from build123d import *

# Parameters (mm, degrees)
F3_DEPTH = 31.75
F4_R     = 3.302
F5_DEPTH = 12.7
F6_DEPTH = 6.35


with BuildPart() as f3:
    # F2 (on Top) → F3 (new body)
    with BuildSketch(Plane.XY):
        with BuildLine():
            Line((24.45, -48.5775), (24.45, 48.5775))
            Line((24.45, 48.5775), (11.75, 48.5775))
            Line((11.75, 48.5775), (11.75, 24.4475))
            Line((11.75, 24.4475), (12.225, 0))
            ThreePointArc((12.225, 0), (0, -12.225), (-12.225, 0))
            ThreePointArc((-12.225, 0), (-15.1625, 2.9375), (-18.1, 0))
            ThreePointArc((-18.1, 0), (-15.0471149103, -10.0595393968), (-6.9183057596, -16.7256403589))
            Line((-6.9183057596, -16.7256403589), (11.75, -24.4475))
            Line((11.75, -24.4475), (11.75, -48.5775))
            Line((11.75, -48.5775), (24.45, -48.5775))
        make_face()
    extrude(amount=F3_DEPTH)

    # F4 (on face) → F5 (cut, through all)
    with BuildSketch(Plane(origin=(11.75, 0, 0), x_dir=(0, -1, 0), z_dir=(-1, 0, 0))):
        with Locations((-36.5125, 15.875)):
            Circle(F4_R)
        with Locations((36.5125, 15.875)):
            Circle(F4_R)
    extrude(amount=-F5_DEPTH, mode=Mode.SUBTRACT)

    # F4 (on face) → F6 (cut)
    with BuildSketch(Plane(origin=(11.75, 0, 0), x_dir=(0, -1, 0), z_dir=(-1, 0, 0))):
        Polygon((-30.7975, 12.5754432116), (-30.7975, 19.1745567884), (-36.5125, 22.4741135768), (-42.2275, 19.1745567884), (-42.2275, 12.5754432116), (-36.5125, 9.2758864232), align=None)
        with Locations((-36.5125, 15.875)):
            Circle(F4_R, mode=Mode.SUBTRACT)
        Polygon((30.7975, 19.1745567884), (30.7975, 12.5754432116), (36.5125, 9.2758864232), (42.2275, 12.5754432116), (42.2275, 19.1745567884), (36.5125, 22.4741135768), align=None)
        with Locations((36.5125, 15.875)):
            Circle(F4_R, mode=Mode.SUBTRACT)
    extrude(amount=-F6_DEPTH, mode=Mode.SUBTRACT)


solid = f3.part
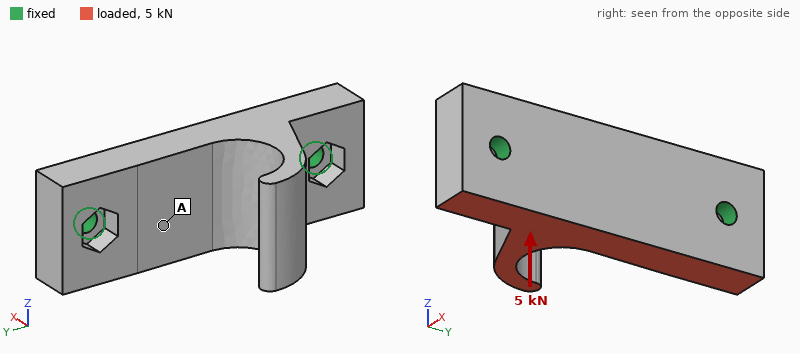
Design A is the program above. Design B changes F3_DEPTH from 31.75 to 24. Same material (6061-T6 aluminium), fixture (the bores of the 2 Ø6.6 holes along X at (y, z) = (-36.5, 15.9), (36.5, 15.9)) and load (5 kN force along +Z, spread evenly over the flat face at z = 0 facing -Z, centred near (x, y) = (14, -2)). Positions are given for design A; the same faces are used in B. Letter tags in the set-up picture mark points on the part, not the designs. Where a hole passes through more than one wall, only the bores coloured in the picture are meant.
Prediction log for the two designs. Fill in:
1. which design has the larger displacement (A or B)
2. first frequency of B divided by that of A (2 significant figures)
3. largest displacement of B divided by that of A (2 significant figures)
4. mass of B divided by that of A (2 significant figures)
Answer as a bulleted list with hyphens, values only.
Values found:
- B
- 1.0
- 1.3
- 0.75
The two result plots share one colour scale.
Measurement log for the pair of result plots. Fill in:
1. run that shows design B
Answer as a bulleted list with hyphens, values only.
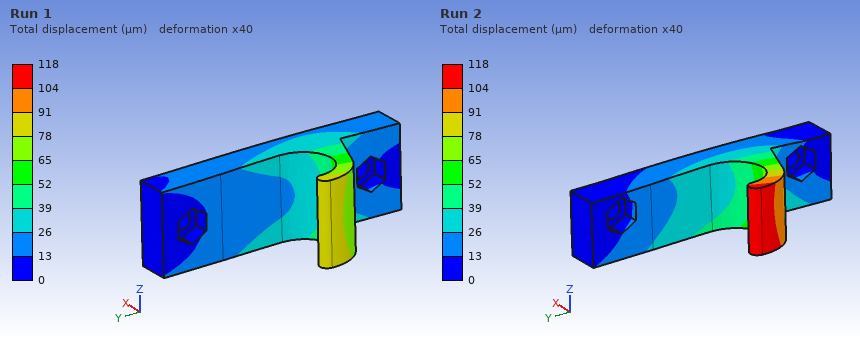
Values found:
- Run 2
